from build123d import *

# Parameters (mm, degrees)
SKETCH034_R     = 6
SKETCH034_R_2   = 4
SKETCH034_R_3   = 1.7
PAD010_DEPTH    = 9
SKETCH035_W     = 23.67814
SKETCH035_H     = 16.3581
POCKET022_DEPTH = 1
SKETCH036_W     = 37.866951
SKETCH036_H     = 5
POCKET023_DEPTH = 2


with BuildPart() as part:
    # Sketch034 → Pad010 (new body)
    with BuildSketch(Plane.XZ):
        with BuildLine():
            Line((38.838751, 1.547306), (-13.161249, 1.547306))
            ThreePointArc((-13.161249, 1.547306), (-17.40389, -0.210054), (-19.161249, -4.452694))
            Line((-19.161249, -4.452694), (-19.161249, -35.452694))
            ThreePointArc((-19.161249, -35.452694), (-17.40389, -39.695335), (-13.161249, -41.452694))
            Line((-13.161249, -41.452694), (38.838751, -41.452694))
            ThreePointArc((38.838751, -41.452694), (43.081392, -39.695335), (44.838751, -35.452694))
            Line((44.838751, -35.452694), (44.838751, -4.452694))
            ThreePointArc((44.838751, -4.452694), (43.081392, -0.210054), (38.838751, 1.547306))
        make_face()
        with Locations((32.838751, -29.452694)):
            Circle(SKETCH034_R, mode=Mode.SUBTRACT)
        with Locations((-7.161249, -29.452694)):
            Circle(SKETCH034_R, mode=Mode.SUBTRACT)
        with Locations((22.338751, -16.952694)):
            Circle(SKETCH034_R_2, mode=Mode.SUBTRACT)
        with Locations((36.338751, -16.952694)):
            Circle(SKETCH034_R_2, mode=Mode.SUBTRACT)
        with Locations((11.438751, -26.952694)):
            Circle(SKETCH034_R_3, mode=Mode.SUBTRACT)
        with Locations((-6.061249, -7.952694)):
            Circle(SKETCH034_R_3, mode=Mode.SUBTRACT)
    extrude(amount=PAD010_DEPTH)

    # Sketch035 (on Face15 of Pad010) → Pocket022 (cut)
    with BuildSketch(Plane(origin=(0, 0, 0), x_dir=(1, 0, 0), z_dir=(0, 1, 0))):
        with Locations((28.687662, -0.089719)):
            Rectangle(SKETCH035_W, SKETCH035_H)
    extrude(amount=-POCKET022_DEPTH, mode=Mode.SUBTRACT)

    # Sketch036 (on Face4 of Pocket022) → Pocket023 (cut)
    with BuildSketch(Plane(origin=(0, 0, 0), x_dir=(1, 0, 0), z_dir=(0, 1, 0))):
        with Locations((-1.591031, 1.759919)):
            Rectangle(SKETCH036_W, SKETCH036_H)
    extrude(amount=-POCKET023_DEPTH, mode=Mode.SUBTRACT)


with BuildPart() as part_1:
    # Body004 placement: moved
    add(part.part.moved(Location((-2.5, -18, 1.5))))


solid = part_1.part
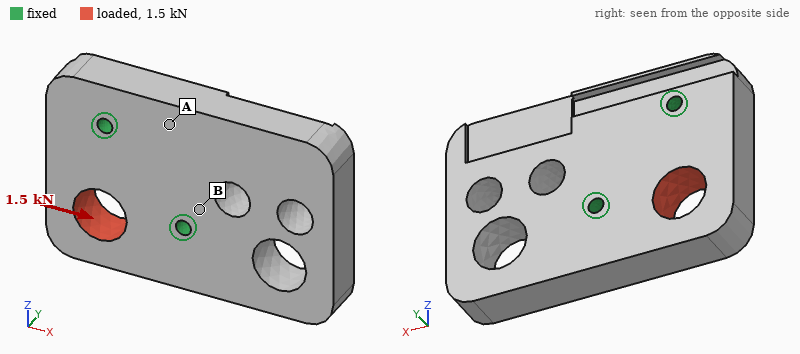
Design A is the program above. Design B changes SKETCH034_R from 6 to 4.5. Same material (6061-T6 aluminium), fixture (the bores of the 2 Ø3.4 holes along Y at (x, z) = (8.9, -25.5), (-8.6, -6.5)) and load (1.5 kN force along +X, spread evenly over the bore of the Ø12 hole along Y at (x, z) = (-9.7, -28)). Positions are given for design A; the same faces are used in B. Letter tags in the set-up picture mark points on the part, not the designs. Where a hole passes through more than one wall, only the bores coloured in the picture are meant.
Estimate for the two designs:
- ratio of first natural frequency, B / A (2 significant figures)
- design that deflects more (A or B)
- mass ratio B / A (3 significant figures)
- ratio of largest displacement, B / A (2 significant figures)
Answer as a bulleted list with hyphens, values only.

- 1.0
- A
- 1.04
- 0.80
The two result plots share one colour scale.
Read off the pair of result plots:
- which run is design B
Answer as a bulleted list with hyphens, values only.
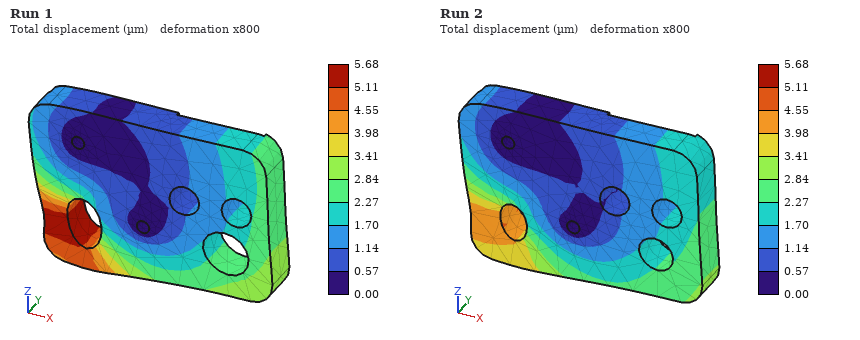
- Run 2
